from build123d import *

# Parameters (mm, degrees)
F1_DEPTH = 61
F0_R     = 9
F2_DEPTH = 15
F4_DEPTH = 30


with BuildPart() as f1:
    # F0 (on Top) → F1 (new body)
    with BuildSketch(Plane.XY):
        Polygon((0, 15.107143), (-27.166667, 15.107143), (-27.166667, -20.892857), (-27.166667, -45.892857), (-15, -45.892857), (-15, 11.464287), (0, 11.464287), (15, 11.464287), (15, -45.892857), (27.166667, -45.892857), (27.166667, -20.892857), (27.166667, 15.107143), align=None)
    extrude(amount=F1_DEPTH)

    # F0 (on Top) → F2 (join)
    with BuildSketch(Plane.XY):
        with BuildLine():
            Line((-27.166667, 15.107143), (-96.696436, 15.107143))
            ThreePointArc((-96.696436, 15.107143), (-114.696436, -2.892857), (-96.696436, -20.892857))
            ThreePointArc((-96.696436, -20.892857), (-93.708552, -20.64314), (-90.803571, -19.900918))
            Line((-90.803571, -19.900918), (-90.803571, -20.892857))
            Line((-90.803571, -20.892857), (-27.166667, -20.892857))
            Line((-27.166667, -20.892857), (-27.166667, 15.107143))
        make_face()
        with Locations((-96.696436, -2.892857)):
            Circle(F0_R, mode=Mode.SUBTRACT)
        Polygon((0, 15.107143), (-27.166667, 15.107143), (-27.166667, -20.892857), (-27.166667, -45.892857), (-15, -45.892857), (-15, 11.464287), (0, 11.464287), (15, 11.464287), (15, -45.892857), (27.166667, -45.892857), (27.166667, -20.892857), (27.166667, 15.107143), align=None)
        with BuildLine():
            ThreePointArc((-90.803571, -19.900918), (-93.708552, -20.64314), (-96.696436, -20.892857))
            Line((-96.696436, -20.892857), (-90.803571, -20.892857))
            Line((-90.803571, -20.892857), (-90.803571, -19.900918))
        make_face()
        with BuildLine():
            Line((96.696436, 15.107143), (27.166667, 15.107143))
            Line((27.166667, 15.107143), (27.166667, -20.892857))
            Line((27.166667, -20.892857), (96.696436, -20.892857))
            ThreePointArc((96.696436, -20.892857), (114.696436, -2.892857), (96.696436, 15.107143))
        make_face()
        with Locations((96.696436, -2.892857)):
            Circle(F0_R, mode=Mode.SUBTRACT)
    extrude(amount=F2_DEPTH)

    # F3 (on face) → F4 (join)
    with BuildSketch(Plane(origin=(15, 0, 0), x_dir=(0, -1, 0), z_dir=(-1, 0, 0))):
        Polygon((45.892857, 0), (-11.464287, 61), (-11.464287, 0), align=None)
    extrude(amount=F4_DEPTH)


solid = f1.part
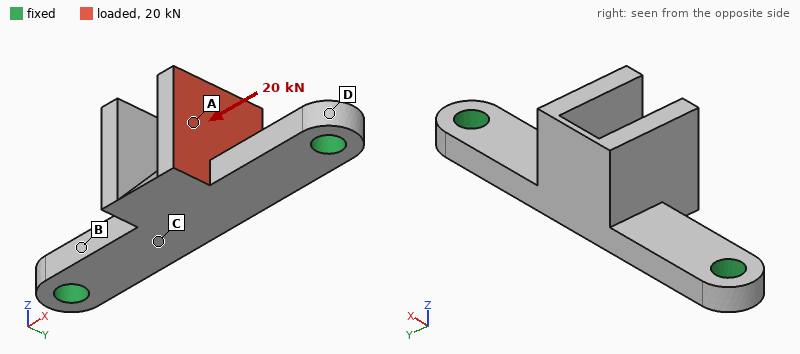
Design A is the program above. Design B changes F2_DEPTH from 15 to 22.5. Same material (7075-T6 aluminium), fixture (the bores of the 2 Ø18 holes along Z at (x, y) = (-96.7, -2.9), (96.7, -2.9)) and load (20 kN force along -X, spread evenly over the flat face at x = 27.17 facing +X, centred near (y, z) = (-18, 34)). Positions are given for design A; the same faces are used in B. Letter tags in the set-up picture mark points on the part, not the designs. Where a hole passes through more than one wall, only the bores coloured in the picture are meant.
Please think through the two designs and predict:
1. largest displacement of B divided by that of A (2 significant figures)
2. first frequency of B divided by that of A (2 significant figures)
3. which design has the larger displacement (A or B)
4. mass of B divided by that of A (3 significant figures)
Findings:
0.70
1.6
A
1.18
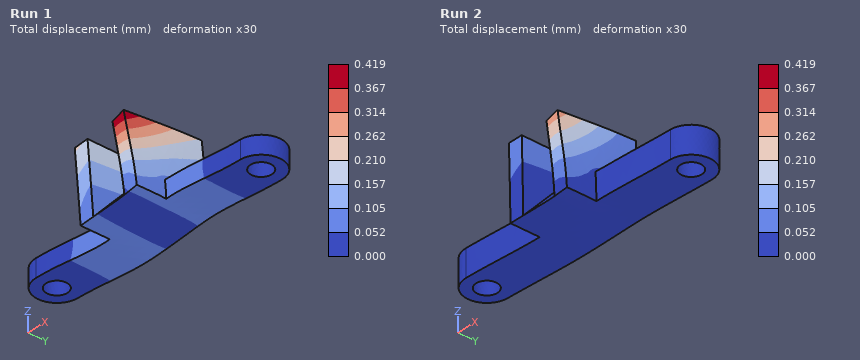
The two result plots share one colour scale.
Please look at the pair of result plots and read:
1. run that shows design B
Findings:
Run 2
